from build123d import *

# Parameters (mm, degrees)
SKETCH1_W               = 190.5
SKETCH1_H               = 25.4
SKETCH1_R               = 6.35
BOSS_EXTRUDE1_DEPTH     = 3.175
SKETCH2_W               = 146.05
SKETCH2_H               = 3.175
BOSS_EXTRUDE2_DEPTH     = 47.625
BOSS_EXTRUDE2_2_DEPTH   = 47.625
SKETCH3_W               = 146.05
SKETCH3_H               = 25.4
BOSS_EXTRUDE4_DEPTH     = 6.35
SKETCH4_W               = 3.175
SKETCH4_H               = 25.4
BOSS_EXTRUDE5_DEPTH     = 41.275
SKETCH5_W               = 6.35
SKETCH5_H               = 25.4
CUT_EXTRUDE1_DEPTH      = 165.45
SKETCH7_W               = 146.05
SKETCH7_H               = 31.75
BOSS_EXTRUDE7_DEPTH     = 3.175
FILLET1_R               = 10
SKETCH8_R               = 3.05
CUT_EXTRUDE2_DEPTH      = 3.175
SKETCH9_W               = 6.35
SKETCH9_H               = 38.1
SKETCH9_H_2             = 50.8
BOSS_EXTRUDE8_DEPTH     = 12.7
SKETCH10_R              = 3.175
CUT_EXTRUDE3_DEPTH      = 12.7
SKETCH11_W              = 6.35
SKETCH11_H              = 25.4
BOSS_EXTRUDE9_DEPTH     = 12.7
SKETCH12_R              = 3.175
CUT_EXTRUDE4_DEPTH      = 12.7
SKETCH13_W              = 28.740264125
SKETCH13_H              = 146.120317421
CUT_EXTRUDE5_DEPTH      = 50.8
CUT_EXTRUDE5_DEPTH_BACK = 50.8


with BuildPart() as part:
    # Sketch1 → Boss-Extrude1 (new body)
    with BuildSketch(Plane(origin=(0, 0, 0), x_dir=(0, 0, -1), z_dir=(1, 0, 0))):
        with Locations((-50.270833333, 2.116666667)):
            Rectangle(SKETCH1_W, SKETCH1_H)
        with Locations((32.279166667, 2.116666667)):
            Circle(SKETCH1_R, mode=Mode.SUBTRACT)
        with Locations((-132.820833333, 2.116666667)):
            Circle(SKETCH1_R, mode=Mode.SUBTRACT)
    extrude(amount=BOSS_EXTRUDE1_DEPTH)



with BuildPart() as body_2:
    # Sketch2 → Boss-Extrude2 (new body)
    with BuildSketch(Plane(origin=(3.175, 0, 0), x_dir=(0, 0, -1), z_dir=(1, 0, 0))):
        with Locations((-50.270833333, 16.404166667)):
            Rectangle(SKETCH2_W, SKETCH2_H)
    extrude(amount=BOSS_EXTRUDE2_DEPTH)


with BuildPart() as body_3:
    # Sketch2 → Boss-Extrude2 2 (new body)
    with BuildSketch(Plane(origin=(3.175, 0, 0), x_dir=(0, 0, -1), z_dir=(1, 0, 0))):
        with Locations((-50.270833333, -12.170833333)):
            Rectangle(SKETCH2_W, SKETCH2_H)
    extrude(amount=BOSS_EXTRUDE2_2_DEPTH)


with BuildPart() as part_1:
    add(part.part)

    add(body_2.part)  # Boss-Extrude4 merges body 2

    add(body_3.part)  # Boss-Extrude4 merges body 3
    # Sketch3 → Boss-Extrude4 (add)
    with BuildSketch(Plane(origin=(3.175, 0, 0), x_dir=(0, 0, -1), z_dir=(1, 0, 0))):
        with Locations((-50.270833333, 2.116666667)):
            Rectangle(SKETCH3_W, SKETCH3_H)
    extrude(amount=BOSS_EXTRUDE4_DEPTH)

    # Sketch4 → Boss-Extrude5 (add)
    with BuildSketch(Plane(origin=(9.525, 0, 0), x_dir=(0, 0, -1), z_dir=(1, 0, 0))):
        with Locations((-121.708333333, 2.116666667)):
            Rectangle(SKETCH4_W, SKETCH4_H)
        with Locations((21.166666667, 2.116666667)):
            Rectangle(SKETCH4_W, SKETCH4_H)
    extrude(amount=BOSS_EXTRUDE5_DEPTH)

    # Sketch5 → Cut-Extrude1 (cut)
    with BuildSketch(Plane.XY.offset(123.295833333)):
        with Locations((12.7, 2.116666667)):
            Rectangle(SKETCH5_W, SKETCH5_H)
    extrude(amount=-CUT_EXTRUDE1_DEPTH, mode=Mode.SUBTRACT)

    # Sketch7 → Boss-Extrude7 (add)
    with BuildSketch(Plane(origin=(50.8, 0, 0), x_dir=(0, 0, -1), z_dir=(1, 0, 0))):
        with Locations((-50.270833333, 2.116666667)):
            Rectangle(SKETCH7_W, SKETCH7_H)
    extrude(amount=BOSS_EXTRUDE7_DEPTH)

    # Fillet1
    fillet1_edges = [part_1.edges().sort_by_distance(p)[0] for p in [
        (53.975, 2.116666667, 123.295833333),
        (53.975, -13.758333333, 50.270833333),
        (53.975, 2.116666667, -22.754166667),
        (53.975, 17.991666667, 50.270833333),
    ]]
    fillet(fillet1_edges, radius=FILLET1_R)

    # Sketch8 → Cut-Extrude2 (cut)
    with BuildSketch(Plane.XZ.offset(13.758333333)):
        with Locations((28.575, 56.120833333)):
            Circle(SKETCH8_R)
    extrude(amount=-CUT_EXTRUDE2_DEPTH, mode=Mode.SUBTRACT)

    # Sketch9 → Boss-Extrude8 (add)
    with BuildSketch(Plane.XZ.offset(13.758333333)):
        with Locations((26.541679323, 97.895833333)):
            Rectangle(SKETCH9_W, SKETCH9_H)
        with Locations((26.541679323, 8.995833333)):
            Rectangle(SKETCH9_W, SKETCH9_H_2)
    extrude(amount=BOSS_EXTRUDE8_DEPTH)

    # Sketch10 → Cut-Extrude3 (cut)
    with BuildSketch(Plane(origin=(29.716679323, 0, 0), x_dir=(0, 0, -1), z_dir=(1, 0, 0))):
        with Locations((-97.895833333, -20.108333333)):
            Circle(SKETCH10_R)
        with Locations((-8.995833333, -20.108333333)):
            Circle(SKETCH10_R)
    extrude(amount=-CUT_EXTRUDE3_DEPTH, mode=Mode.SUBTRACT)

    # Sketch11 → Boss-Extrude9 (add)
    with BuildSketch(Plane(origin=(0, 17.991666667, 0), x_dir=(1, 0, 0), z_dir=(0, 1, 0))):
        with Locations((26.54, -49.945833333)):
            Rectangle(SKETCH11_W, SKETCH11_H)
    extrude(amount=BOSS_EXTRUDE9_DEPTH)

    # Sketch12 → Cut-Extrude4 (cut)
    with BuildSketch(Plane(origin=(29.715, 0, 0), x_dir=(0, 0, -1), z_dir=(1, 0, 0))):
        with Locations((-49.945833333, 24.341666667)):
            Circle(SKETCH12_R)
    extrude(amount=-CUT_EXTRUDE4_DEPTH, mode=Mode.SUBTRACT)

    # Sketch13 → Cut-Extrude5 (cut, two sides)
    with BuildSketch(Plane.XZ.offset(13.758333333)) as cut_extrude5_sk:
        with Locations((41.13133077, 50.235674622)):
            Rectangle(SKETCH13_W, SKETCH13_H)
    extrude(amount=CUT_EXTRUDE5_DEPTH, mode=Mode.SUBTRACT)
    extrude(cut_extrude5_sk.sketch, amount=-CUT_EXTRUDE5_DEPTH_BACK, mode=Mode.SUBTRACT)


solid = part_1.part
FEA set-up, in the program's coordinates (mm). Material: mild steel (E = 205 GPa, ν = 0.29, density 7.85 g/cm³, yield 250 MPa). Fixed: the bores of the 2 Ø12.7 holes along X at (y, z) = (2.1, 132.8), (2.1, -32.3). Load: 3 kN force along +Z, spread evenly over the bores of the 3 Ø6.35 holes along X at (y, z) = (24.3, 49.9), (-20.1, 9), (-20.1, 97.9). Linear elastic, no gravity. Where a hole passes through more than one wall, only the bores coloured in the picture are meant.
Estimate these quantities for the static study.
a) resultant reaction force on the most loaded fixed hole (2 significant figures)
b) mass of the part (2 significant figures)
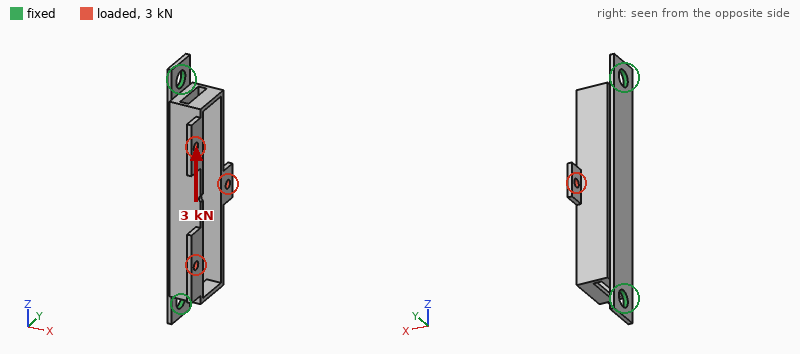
1.6 kN
520 g
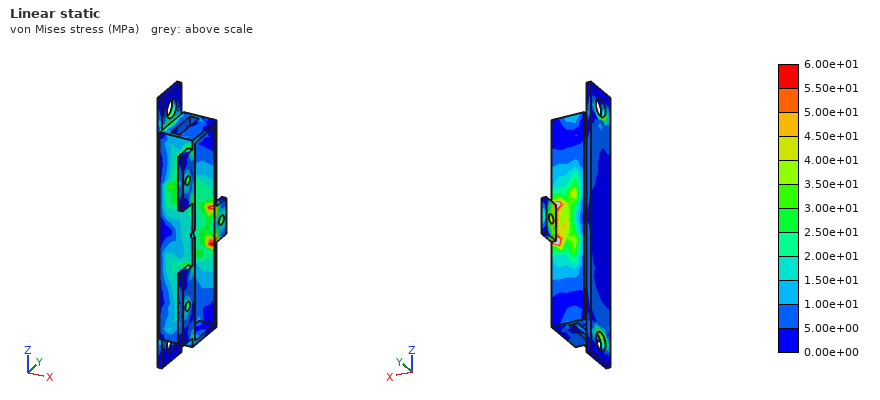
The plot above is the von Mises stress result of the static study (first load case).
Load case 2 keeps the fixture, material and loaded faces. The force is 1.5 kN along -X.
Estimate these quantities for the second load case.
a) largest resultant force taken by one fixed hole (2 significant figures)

1.6 kN
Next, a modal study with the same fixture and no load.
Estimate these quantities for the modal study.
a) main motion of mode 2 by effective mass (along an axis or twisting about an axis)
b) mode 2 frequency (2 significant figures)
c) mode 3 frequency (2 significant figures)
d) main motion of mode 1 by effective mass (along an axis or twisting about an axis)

along X
2500 Hz
3300 Hz
along Y
